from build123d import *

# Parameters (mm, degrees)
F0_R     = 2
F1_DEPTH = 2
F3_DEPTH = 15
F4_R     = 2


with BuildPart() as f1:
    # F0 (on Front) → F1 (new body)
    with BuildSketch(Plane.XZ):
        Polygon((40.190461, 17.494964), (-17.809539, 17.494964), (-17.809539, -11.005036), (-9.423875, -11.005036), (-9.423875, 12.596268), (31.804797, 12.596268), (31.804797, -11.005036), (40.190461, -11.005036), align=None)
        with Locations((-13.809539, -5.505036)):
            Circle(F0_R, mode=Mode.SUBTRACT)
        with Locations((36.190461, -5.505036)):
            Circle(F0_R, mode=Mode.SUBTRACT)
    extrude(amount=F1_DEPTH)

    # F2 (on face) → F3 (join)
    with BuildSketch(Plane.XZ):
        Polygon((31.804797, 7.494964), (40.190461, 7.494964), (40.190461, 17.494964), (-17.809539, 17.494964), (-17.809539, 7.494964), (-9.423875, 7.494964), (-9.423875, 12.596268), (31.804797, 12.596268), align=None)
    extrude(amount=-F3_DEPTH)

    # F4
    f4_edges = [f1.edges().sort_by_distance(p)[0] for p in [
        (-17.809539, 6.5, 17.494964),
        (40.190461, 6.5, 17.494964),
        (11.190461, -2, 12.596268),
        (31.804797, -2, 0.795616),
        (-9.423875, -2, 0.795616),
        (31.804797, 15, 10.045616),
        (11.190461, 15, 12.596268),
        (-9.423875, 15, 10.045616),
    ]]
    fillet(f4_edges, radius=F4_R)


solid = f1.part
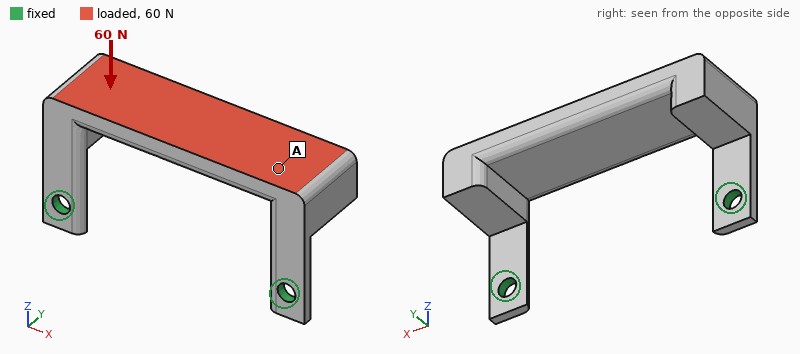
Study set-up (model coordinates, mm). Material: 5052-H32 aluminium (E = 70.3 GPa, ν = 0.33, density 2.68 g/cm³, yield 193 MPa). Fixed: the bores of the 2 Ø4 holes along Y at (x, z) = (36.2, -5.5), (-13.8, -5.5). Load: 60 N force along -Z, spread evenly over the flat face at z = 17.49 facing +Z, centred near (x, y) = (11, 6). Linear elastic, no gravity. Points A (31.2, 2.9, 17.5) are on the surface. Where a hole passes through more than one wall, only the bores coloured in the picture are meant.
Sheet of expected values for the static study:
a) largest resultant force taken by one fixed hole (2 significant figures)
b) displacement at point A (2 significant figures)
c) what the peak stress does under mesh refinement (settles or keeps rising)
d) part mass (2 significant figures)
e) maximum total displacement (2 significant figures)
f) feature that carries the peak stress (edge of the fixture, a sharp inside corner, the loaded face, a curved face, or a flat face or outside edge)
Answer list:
31 N
0.12 mm
keeps rising
18 g
0.17 mm
edge of the fixture
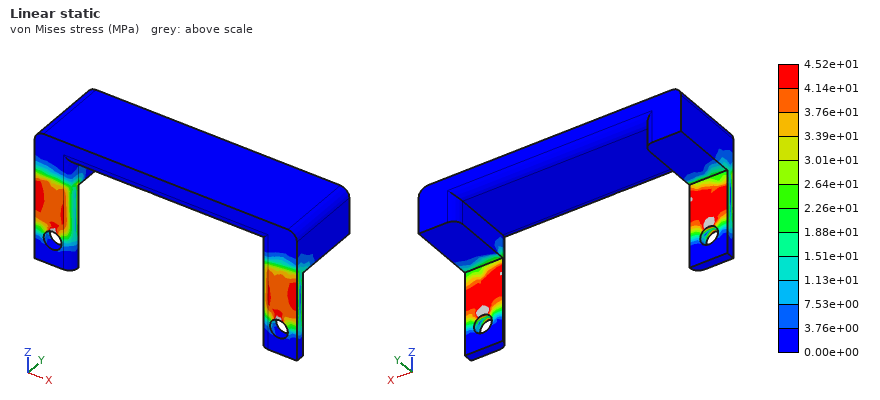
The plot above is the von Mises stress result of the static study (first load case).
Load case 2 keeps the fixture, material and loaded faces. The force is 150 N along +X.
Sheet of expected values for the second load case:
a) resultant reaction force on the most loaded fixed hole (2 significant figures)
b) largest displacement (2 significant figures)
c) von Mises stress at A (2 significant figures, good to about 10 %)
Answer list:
87 N
24 µm
7.9 MPa
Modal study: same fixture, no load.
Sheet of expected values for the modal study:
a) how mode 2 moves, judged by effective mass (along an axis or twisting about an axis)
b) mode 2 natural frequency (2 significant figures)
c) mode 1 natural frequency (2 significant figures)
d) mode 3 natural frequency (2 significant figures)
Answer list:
along X
2600 Hz
630 Hz
4000 Hz
